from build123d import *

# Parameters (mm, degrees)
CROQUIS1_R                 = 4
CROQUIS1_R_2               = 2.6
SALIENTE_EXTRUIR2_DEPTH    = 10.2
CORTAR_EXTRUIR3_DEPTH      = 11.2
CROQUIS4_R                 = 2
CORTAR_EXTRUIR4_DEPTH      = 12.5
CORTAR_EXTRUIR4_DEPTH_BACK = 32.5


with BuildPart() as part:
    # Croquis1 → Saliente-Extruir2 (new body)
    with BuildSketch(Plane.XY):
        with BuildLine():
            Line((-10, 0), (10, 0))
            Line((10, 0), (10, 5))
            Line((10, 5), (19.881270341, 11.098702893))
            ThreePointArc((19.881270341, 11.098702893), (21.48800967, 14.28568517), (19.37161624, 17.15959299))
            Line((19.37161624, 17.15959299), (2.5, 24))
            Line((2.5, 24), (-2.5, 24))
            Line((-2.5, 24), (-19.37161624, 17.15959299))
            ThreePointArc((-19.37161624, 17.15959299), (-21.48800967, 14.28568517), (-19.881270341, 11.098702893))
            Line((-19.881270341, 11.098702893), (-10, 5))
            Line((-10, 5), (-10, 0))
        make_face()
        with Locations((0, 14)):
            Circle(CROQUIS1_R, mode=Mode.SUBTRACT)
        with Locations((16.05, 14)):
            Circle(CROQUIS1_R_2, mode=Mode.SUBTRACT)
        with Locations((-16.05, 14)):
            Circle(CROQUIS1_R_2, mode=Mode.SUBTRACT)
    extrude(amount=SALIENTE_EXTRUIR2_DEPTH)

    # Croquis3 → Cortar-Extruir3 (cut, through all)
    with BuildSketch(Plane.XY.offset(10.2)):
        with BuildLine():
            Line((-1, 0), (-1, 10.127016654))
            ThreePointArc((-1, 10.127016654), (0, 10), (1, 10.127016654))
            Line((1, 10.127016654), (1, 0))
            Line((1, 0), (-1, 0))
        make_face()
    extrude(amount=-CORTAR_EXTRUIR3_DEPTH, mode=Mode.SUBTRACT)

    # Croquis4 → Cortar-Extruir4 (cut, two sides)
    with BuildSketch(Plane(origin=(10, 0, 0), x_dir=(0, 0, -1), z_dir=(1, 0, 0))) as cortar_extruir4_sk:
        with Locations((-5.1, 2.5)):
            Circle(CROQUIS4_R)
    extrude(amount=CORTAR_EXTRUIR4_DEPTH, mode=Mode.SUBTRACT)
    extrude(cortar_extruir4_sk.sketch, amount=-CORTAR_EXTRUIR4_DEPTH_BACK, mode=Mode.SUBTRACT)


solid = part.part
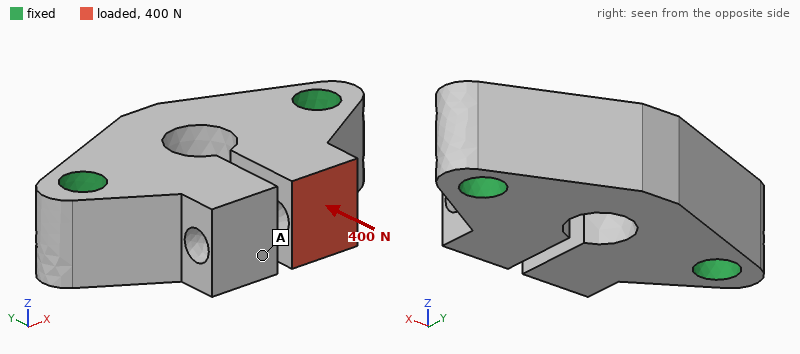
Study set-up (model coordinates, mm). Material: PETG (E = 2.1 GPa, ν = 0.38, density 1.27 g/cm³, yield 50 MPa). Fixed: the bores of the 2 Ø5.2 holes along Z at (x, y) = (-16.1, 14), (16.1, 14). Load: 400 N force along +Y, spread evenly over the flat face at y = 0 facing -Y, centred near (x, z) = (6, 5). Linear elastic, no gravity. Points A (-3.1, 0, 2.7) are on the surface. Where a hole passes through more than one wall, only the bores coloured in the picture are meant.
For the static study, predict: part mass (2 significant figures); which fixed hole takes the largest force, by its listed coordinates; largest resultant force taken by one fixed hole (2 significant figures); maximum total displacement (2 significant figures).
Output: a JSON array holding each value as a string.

["7.1 g", "(16.1, 14)", "340 N", "0.23 mm"]
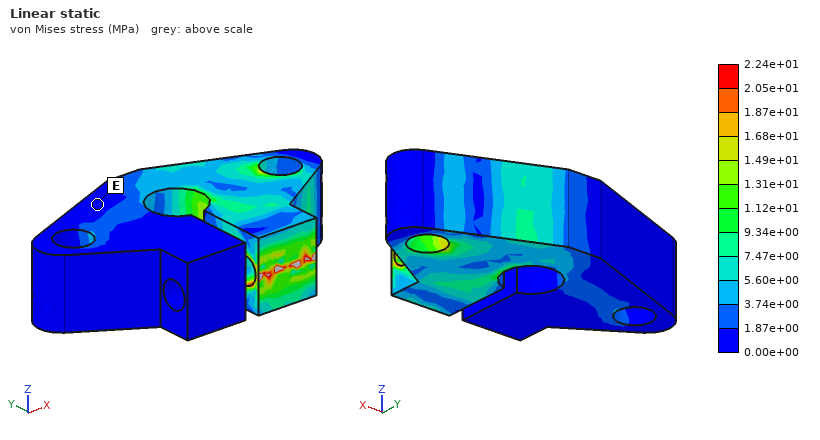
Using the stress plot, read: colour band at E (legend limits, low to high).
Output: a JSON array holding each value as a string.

["0.00e+00 to 1.87e+00 MPa"]
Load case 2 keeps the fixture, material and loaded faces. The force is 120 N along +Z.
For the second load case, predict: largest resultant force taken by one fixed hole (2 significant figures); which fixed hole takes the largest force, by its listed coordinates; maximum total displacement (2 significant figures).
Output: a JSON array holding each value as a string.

["120 N", "(16.1, 14)", "0.19 mm"]
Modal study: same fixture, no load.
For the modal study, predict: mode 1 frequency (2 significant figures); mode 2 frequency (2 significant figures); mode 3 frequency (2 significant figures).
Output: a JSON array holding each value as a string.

["6200 Hz", "6200 Hz", "6400 Hz"]
